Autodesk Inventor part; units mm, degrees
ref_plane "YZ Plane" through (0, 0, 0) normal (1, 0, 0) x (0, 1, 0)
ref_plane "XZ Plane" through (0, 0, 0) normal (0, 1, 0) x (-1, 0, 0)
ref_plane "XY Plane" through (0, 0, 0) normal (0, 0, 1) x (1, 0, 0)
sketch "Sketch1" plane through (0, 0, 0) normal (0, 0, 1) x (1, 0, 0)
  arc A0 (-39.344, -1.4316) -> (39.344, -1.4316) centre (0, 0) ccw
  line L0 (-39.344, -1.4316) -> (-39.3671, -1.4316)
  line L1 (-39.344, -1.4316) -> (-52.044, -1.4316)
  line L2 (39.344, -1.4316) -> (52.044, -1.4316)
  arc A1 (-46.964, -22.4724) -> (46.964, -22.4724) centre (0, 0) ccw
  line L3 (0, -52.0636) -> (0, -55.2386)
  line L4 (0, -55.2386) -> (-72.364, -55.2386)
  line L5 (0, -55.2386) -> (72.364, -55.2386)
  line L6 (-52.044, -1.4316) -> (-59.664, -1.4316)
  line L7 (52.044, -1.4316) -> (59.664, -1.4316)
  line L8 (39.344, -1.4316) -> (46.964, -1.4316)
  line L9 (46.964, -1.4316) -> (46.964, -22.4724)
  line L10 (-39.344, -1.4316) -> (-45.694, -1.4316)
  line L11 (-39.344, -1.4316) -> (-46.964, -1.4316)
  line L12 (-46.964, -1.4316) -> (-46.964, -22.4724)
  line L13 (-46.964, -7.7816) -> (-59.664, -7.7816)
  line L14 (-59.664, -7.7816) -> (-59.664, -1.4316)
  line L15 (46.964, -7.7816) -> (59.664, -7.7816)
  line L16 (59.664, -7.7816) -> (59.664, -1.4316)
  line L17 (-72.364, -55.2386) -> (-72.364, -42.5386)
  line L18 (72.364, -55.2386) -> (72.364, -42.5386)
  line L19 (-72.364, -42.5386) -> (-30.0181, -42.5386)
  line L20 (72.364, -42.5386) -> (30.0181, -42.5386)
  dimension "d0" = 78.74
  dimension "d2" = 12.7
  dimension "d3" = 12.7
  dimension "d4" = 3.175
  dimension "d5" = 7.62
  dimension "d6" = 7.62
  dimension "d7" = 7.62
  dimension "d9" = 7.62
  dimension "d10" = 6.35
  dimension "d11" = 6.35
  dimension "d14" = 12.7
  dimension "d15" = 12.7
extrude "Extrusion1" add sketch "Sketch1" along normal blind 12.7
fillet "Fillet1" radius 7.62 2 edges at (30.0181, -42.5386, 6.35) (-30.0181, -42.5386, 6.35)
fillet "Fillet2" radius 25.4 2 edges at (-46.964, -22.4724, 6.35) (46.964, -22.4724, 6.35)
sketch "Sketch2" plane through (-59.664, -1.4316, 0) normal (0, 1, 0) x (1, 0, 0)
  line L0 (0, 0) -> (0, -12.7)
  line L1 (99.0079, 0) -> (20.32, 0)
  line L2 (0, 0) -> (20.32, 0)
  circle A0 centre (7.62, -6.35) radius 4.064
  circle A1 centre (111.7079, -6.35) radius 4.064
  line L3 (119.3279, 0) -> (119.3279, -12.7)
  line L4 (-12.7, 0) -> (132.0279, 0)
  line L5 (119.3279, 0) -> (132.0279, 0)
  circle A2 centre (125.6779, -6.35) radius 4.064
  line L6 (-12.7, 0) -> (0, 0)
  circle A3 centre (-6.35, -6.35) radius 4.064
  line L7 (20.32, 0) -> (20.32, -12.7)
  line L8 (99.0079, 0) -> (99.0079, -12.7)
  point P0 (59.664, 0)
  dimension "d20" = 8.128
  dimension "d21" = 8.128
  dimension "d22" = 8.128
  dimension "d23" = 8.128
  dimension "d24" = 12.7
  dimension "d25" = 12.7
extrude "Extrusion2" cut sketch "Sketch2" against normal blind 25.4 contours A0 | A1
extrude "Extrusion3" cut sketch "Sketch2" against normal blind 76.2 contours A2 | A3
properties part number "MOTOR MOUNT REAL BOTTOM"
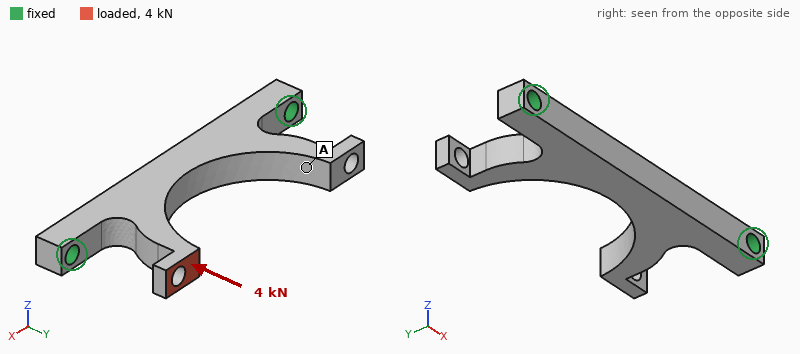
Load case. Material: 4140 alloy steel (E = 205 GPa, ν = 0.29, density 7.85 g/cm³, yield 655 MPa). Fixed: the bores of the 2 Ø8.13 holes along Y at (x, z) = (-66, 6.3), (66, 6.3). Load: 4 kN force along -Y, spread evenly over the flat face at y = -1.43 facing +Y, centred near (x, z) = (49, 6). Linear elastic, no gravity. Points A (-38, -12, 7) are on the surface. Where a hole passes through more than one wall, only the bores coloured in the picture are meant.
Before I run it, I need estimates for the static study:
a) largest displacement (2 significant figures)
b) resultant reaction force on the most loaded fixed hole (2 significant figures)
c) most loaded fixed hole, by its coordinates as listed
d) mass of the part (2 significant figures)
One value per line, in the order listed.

0.18 mm
3.9 kN
(66, 6.3)
320 g
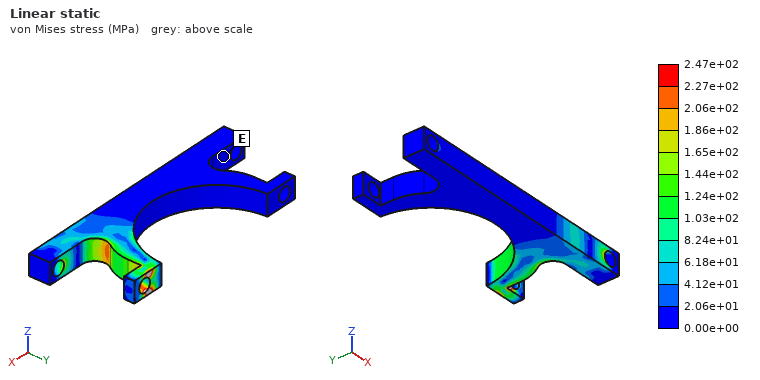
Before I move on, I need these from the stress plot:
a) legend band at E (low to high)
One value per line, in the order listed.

0.00e+00 to 2.06e+01 MPa
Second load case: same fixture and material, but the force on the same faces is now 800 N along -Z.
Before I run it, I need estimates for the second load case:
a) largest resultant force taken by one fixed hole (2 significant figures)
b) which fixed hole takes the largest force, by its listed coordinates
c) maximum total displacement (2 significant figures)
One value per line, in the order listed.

790 N
(66, 6.3)
0.17 mm
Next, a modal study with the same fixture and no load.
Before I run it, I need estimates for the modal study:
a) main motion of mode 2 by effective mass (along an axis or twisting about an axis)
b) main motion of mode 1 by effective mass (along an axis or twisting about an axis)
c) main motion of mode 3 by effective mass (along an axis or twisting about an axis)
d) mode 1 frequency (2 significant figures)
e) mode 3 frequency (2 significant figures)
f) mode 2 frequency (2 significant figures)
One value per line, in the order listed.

twisting about Y
along Z
along Y
2100 Hz
3300 Hz
3100 Hz
